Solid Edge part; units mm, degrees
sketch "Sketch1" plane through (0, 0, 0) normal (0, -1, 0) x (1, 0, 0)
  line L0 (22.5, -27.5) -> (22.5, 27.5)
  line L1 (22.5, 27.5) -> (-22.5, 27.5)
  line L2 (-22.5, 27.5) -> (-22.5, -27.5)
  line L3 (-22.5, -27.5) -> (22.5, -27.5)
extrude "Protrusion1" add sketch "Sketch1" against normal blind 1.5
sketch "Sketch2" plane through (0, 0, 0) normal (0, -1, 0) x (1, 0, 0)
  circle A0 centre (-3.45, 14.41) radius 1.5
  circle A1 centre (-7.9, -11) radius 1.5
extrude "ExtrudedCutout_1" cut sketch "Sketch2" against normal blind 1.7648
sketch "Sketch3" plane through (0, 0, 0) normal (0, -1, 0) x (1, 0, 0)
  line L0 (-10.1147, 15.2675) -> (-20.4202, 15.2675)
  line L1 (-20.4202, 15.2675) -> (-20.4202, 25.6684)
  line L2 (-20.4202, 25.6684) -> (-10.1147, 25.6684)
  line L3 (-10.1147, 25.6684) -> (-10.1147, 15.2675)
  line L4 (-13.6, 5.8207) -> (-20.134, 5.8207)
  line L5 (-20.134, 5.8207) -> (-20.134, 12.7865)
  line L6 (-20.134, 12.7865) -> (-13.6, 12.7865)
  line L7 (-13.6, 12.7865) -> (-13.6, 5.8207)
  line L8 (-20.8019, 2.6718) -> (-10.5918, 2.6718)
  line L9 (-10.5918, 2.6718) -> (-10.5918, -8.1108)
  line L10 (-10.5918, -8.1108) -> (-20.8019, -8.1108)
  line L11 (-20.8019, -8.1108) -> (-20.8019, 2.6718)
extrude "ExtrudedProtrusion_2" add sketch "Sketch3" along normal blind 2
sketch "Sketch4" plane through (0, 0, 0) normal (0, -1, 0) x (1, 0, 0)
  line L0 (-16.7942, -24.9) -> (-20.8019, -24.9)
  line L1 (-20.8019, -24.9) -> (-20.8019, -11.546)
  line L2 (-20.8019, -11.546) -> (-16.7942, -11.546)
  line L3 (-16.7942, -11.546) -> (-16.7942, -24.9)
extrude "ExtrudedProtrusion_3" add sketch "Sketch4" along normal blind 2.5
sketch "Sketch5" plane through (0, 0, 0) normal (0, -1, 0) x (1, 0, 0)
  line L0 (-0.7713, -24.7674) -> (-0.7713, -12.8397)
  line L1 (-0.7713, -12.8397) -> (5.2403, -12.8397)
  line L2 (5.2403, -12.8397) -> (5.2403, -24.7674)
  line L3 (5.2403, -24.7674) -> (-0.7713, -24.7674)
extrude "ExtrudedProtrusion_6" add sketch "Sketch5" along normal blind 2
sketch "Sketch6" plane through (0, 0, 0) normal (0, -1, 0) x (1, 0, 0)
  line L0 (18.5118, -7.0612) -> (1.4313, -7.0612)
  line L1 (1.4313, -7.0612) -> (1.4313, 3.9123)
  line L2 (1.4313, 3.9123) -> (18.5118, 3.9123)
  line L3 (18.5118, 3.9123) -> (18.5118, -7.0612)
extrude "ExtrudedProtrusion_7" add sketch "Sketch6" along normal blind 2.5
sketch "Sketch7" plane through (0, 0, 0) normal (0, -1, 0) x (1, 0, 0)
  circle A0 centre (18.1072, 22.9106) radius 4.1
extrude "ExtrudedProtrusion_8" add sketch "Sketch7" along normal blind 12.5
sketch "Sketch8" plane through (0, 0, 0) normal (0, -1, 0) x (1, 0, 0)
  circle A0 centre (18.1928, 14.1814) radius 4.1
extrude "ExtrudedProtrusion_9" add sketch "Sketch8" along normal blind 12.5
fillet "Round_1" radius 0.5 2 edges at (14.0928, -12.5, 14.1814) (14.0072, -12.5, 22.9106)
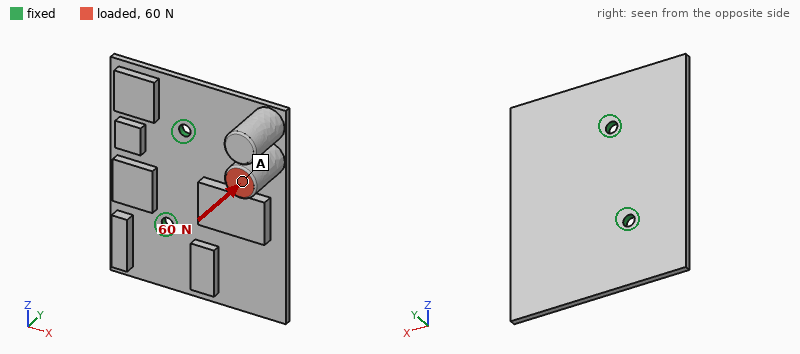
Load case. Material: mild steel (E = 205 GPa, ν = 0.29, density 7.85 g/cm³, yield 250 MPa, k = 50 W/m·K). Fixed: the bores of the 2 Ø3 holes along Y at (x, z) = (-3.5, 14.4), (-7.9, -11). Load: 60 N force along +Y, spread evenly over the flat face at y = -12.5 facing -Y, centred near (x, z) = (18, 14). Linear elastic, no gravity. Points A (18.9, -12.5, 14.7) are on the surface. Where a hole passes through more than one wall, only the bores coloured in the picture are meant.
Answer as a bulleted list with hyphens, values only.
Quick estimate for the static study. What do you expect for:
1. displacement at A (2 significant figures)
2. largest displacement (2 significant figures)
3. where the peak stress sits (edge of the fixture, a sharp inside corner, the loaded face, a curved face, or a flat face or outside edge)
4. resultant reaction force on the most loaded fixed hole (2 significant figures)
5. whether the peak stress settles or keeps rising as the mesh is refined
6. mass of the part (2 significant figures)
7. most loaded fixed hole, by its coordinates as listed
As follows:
- 0.10 mm
- 0.12 mm
- edge of the fixture
- 64 N
- keeps rising
- 49 g
- (-3.5, 14.4)
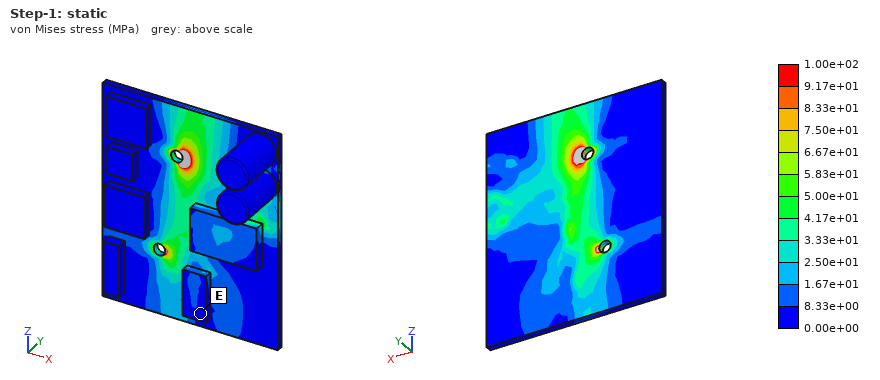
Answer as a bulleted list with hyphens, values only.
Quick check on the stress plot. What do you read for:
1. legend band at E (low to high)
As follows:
- 0.00e+00 to 8.33e+00 MPa
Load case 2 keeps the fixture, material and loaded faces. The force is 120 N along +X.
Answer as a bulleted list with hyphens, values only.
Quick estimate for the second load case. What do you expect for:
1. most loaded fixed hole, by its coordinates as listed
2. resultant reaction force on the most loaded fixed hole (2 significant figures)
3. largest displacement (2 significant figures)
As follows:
- (-3.5, 14.4)
- 110 N
- 0.22 mm
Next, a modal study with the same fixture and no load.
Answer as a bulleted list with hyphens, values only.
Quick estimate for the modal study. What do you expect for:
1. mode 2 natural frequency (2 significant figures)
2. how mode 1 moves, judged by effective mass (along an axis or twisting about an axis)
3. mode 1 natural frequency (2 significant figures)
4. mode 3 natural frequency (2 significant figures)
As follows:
- 1700 Hz
- along Y
- 950 Hz
- 3000 Hz
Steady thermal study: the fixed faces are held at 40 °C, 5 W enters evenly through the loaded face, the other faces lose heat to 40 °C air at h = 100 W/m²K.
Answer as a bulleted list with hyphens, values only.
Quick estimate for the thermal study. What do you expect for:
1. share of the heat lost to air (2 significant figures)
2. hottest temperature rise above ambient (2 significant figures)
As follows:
- 75 %
- 45 K
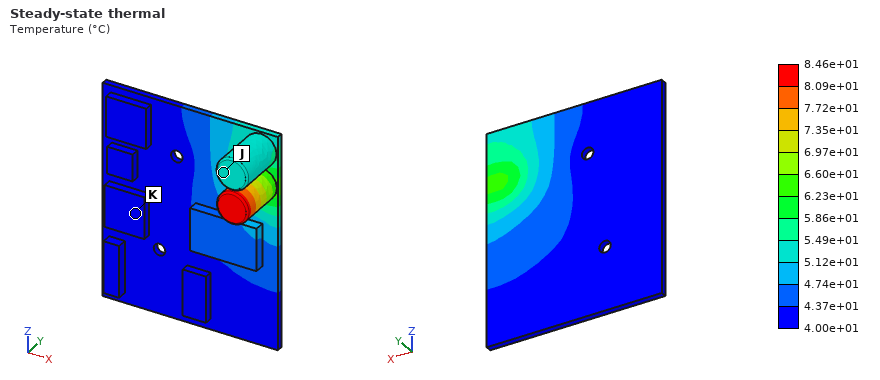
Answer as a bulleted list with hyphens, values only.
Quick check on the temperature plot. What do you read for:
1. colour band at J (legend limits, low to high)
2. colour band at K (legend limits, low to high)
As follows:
- 5.12e+01 to 5.49e+01 °C
- 4.00e+01 to 4.37e+01 °C
